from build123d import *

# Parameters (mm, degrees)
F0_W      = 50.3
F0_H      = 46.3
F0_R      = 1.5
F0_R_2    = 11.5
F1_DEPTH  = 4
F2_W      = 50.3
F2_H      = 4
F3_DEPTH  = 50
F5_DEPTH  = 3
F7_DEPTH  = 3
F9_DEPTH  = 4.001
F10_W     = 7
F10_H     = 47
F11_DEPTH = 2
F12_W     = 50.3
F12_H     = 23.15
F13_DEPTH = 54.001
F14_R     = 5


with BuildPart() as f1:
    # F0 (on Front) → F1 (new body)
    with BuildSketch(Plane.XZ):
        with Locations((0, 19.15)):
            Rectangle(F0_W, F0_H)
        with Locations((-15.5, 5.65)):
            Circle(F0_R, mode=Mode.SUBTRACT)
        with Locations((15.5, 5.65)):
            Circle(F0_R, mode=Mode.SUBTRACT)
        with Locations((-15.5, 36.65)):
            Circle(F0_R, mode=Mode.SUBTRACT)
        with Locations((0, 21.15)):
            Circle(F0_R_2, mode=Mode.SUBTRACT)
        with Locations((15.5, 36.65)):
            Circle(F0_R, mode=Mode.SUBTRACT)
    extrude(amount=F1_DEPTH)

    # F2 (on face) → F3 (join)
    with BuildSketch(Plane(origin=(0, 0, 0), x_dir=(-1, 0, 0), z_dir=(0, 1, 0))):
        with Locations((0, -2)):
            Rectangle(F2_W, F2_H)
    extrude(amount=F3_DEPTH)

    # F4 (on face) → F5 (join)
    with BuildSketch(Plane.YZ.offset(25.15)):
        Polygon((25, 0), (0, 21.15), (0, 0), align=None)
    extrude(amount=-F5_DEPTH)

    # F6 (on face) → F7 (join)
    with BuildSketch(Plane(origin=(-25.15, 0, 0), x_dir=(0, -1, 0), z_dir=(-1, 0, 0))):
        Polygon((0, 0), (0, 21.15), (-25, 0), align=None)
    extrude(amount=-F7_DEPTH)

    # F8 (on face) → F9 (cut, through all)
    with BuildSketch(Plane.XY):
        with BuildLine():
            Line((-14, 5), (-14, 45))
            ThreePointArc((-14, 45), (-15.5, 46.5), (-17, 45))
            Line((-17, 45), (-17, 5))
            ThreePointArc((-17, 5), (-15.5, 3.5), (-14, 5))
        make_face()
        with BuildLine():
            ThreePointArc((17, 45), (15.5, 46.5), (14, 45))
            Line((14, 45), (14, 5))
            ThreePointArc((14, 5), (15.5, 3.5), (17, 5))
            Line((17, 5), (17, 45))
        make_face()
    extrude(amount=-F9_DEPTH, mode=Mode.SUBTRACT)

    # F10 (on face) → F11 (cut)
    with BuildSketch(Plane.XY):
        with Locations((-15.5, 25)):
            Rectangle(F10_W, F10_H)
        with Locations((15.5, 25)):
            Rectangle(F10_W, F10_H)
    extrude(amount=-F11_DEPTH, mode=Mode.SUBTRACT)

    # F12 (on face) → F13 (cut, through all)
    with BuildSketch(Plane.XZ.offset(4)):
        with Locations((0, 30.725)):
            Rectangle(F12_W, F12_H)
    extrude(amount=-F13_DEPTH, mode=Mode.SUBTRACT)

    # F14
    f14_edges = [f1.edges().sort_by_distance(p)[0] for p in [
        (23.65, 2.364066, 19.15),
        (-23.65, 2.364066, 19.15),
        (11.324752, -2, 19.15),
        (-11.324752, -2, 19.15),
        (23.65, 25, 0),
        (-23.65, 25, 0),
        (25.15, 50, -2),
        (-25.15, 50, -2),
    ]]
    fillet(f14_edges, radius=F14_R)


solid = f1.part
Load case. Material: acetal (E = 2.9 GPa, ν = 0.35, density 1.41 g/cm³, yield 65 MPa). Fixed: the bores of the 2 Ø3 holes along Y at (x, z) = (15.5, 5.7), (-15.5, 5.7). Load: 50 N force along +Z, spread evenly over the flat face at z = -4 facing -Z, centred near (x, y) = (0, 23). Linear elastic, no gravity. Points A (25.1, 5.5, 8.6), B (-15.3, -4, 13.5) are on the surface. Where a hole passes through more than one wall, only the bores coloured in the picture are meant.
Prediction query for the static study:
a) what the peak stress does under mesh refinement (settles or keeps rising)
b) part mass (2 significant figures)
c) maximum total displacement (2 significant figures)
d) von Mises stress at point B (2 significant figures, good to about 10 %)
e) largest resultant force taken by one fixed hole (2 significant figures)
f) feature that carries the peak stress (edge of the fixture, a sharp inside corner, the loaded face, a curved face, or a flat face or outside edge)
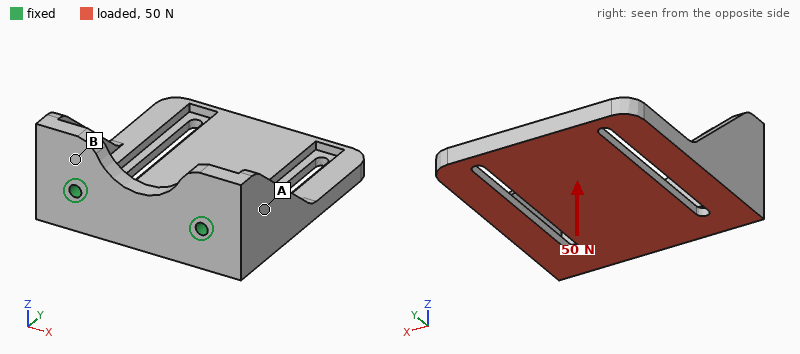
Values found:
keeps rising
19 g
0.92 mm
3.2 MPa
26 N
edge of the fixture
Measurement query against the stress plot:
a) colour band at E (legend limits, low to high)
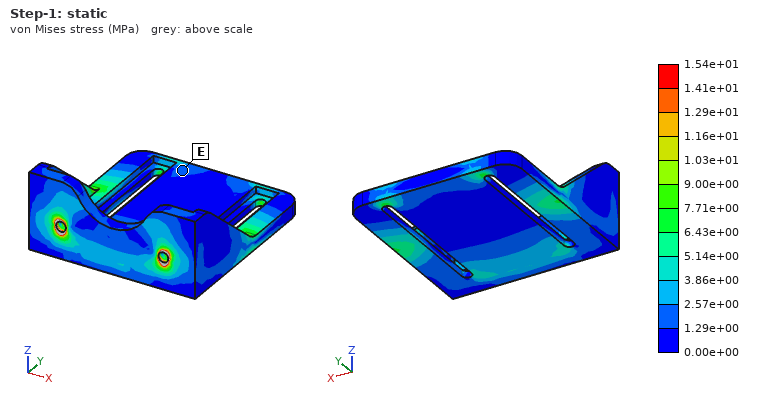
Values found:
1.29e+00 to 2.57e+00 MPa
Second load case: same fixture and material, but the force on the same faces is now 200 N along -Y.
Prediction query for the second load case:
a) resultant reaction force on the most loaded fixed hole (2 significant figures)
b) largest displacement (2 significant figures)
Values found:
100 N
0.81 mm
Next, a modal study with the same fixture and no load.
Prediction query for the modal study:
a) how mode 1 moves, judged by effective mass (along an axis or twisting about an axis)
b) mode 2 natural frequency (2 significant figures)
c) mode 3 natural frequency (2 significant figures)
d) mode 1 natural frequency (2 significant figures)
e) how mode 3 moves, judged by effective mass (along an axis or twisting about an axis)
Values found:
along Z
870 Hz
1300 Hz
410 Hz
along X
